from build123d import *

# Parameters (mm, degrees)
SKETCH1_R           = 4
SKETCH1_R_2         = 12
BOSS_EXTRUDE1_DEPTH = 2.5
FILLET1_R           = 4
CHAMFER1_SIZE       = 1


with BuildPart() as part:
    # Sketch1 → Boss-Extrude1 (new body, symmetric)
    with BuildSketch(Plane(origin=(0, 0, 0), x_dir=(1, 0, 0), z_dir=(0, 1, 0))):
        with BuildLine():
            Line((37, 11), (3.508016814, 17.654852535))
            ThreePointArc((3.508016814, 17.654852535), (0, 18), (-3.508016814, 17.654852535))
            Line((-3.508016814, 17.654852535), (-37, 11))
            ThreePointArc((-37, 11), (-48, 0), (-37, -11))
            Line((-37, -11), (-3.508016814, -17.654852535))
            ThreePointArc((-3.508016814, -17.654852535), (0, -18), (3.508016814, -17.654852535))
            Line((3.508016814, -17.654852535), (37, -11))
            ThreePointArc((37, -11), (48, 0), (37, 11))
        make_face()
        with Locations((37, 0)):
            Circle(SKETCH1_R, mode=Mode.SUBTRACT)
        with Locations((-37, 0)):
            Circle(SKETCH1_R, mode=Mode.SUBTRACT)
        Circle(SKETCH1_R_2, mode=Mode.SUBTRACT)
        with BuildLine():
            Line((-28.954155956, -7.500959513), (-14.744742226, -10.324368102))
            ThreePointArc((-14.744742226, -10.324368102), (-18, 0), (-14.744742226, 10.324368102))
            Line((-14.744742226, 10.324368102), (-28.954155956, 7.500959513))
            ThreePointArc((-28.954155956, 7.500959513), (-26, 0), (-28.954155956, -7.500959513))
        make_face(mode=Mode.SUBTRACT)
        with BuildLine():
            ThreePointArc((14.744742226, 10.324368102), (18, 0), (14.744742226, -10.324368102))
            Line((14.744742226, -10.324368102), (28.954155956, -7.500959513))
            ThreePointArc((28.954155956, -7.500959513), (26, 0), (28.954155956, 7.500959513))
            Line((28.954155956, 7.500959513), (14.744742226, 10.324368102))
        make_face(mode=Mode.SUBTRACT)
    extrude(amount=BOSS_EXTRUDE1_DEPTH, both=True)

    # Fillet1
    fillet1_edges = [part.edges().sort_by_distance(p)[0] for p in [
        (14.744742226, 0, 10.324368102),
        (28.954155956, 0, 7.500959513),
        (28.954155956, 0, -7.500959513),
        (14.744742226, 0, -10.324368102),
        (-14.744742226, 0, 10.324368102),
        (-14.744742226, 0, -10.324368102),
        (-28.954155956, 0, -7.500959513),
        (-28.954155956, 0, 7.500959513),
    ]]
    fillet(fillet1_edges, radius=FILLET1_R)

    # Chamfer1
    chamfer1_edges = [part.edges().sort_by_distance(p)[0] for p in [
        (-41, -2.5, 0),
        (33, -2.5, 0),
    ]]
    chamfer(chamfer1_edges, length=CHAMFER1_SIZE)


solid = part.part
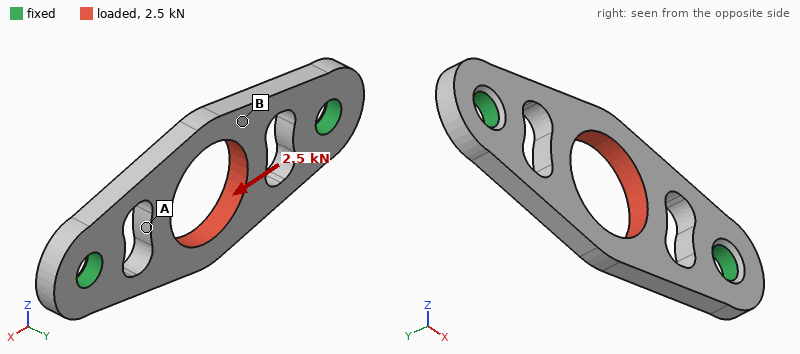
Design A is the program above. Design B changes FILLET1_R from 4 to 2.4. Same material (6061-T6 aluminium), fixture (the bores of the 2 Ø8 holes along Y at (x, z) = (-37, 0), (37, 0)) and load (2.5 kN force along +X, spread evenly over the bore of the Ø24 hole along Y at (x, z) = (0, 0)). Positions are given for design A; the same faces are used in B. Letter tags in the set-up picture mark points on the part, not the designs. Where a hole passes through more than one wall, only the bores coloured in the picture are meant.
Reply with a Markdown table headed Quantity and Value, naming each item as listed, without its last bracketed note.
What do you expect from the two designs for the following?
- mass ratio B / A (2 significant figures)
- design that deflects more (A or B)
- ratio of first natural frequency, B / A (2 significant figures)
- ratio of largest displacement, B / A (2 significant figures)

| Quantity | Value |
|---|---|
| mass ratio B / A | 0.98 |
| design that deflects more | B |
| ratio of first natural frequency, B / A | 0.98 |
| ratio of largest displacement, B / A | 1.1 |
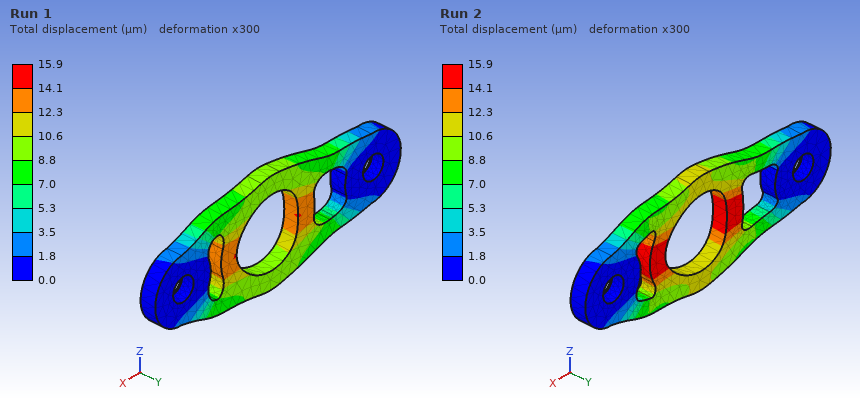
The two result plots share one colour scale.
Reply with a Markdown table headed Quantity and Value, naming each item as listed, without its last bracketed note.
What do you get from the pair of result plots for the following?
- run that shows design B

| Quantity | Value |
|---|---|
| run that shows design B | Run 2 |
